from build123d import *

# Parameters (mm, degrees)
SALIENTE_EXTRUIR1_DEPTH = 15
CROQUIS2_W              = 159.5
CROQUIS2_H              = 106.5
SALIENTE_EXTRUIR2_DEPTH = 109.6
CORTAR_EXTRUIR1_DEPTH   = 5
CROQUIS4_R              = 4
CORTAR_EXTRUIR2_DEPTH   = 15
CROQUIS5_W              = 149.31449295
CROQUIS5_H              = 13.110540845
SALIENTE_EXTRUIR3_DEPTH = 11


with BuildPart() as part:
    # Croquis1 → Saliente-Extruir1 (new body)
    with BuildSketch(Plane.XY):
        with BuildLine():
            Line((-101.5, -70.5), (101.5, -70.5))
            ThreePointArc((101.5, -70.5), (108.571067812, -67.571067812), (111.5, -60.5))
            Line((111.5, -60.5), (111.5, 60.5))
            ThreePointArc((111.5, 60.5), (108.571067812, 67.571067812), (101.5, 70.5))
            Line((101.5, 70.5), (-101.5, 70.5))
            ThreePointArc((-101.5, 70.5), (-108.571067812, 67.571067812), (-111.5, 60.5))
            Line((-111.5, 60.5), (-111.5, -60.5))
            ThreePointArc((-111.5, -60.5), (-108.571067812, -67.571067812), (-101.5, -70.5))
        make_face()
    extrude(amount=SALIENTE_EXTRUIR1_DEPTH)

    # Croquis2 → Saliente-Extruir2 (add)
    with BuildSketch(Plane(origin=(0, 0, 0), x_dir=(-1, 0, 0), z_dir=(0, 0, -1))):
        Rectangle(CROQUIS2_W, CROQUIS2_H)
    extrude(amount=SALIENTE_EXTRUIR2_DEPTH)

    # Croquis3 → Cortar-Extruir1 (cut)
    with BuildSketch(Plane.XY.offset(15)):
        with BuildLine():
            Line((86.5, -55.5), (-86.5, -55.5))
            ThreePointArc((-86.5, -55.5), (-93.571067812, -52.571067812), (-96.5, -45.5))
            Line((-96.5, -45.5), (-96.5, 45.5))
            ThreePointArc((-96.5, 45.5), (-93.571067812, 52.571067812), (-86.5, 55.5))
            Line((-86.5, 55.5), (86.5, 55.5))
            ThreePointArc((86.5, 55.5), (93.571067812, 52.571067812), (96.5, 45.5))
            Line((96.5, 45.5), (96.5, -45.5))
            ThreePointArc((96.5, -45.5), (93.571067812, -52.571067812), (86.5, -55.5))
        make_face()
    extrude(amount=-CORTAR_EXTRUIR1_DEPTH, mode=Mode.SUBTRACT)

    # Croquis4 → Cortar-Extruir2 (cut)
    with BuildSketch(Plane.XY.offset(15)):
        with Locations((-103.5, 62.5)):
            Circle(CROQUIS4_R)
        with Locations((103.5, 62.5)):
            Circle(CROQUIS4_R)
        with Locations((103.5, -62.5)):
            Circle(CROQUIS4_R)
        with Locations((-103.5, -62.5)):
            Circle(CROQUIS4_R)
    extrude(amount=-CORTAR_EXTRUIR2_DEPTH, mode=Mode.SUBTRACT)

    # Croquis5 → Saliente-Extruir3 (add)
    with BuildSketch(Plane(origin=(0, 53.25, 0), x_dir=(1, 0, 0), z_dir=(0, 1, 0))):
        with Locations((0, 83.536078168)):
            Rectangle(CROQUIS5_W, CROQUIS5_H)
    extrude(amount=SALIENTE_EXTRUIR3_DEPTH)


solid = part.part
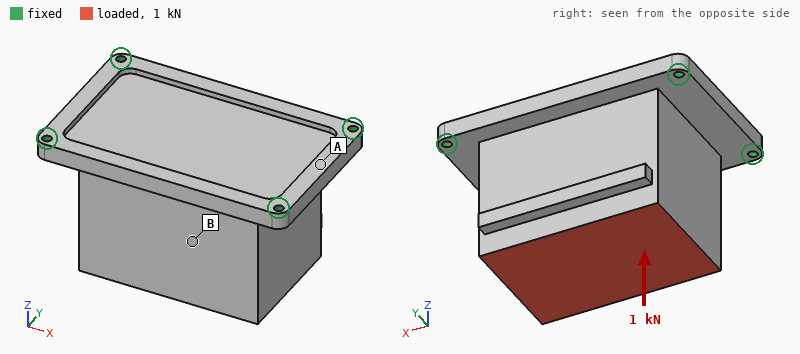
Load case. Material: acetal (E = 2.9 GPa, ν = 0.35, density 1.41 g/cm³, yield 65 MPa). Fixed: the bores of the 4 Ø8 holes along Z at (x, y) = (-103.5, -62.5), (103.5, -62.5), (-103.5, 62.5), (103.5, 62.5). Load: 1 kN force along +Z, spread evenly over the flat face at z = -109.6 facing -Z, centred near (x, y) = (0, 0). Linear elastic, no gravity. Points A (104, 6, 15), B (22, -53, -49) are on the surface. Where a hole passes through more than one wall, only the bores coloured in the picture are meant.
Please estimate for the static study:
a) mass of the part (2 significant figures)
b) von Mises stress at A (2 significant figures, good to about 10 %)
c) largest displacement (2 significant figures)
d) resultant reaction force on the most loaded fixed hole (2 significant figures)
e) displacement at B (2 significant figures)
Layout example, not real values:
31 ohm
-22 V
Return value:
3.2 kg
0.79 MPa
74 µm
300 N
72 µm
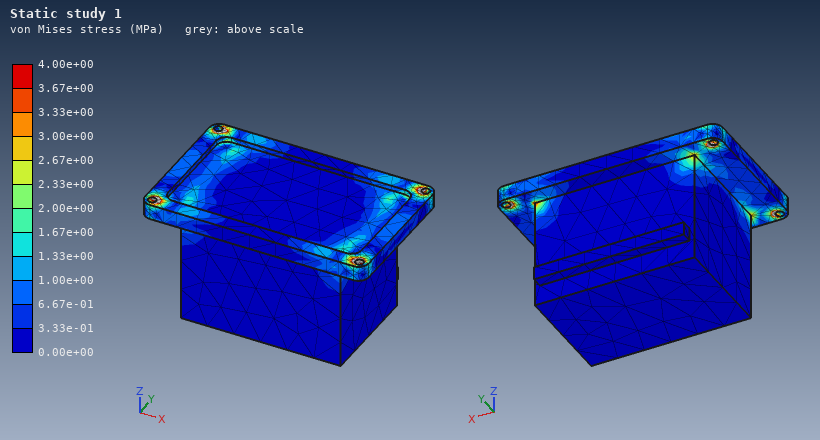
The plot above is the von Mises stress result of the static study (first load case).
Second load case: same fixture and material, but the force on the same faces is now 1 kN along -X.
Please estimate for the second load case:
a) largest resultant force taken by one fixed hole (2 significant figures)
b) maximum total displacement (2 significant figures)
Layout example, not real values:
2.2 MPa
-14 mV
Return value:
430 N
0.15 mm
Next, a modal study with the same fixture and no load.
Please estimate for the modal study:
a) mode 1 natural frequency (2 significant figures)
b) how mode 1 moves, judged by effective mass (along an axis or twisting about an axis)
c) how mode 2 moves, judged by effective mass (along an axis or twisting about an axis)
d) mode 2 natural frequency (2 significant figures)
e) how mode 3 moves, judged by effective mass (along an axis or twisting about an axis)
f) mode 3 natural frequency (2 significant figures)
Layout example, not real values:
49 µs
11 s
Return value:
260 Hz
along Y
along Z
340 Hz
along X
380 Hz
